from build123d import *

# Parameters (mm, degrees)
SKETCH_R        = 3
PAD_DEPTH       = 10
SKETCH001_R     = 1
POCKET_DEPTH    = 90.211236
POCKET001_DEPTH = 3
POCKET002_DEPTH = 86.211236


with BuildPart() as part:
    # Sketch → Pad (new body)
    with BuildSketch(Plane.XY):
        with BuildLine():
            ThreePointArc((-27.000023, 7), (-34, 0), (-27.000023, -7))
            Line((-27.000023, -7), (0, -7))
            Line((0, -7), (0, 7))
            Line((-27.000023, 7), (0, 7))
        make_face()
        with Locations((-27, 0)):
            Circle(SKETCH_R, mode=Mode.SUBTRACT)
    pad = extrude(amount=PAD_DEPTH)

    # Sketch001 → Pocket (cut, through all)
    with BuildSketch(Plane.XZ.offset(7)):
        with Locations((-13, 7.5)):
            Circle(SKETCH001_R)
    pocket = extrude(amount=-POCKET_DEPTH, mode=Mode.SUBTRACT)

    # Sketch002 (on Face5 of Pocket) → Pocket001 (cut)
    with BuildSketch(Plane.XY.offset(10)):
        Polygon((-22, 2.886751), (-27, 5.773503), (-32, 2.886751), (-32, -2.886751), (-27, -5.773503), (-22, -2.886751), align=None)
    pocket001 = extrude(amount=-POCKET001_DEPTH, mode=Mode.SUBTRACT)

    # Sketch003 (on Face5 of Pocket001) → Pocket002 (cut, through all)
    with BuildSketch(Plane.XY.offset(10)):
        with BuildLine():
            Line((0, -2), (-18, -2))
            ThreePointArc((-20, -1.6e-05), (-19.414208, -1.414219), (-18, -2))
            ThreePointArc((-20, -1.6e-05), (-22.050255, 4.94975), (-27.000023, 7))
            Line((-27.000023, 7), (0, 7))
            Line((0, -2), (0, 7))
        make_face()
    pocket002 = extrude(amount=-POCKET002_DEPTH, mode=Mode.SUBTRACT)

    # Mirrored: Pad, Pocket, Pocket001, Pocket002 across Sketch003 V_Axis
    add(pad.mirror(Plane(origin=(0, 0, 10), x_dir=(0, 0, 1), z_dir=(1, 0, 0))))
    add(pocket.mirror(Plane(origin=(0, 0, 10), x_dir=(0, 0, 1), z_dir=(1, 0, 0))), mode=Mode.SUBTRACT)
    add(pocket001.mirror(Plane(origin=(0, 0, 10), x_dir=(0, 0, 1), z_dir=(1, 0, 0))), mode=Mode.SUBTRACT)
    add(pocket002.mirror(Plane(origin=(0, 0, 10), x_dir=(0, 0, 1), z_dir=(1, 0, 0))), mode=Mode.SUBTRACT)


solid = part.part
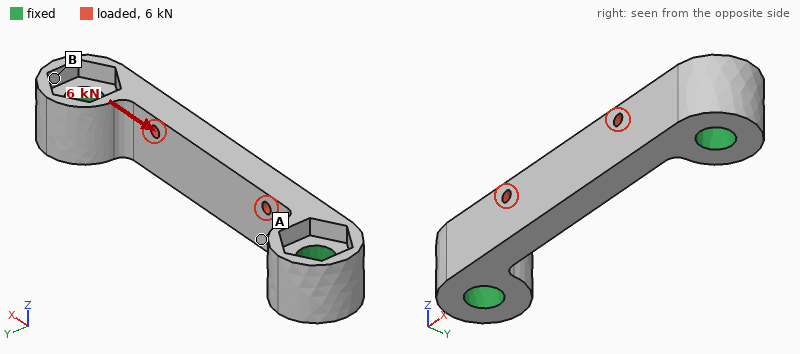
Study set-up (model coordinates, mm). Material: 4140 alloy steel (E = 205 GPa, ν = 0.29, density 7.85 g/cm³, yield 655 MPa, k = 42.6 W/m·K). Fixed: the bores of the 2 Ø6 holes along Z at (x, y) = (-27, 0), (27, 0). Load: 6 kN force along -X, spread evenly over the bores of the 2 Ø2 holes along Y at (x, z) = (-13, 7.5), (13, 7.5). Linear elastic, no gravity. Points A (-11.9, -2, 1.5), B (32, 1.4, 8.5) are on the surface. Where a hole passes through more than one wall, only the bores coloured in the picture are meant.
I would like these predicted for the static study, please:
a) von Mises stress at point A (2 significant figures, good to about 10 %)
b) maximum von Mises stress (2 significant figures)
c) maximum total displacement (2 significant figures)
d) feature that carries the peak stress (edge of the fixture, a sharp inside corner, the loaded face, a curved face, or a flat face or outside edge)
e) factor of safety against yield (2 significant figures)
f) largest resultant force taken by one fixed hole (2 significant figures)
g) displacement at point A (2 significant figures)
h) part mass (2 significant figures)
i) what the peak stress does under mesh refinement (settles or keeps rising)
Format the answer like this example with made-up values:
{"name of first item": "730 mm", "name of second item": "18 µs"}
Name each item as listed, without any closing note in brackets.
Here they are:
{"von Mises stress at point A": "57 MPa", "maximum von Mises stress": "200 MPa", "maximum total displacement": "7.3 µm", "feature that carries the peak stress": "the loaded face", "factor of safety against yield": "3.2", "largest resultant force taken by one fixed hole": "3.0 kN", "displacement at point A": "4.9 µm", "part mass": "34 g", "what the peak stress does under mesh refinement": "settles"}
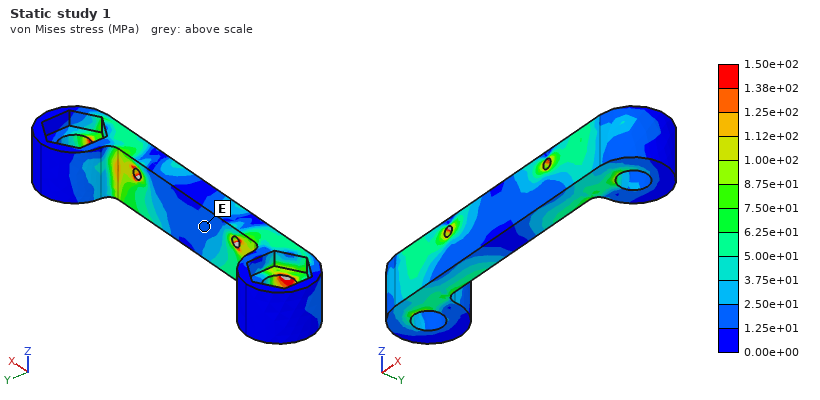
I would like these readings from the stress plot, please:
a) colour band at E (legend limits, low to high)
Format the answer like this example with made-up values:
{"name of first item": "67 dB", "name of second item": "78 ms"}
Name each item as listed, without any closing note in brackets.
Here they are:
{"colour band at E": "1.25e+01 to 2.50e+01 MPa"}
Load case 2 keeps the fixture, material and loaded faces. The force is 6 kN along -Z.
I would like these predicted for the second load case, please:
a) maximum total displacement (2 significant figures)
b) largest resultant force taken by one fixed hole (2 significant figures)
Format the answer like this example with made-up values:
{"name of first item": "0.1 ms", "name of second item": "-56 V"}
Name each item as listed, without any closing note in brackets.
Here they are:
{"maximum total displacement": "42 µm", "largest resultant force taken by one fixed hole": "3.1 kN"}
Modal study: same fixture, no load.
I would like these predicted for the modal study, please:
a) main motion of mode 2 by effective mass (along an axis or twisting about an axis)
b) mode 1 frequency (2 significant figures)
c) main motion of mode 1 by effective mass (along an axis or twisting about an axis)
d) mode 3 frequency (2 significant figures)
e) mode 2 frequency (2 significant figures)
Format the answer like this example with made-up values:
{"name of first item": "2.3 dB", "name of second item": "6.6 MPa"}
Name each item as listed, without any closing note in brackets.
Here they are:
{"main motion of mode 2 by effective mass": "along Z", "mode 1 frequency": "12 kHz", "main motion of mode 1 by effective mass": "along Y", "mode 3 frequency": "27 kHz", "mode 2 frequency": "15 kHz"}
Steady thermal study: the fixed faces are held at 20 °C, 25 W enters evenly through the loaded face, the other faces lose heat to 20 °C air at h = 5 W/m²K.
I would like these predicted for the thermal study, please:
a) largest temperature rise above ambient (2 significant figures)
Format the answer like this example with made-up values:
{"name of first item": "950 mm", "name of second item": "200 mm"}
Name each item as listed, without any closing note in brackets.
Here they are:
{"largest temperature rise above ambient": "82 K"}
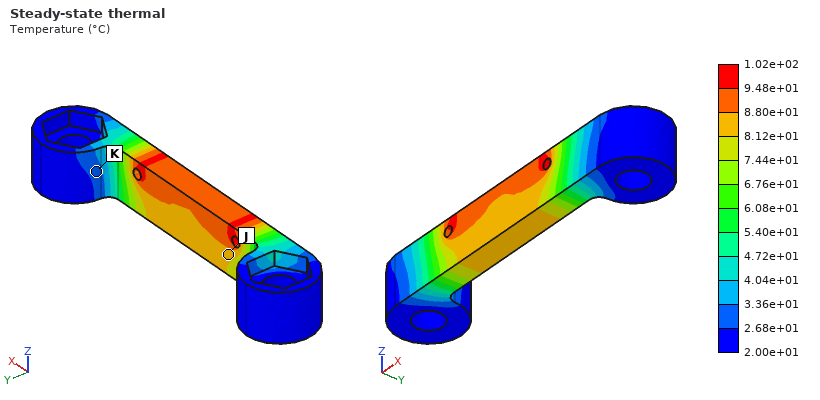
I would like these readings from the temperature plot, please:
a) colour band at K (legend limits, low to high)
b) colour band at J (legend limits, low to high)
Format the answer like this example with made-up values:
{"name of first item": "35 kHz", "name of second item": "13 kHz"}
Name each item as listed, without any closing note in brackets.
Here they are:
{"colour band at K": "2.68e+01 to 3.36e+01 °C", "colour band at J": "8.12e+01 to 8.80e+01 °C"}
